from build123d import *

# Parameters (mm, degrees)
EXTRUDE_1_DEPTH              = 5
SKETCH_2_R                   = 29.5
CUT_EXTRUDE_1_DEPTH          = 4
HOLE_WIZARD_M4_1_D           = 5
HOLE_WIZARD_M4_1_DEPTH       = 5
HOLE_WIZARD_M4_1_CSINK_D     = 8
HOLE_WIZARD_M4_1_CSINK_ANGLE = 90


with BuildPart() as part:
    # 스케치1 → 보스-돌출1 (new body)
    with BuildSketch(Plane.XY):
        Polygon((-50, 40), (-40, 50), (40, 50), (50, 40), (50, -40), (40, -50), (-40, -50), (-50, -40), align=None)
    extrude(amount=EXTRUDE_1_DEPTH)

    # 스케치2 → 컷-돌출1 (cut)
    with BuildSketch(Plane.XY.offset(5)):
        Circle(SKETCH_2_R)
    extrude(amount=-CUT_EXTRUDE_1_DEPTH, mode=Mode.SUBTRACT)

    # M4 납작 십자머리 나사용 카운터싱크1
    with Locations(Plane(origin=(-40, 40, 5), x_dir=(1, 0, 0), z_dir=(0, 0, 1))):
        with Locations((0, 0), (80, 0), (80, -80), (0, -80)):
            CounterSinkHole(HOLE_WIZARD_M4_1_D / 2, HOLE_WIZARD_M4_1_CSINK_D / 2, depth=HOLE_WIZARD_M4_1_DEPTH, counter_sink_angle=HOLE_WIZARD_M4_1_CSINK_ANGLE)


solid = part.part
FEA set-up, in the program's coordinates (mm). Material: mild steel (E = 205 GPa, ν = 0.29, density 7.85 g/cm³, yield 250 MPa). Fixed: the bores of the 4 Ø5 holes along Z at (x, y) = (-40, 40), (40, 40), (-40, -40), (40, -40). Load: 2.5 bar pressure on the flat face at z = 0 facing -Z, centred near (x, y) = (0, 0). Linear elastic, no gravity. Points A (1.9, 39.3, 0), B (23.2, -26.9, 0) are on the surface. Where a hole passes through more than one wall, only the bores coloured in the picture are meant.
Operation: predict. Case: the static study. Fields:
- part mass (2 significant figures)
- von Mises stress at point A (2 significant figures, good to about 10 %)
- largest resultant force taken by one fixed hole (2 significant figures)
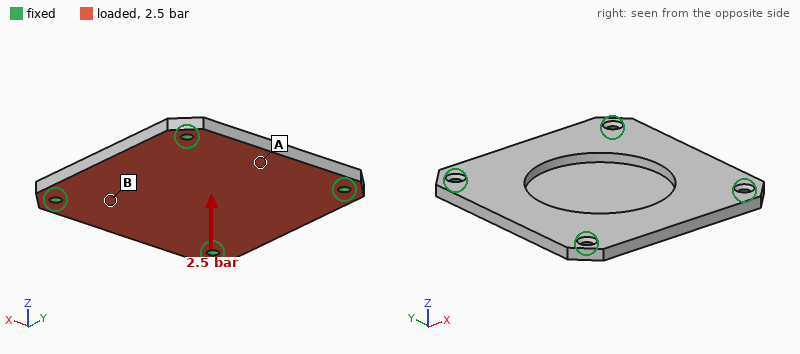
300 g
25 MPa
640 N
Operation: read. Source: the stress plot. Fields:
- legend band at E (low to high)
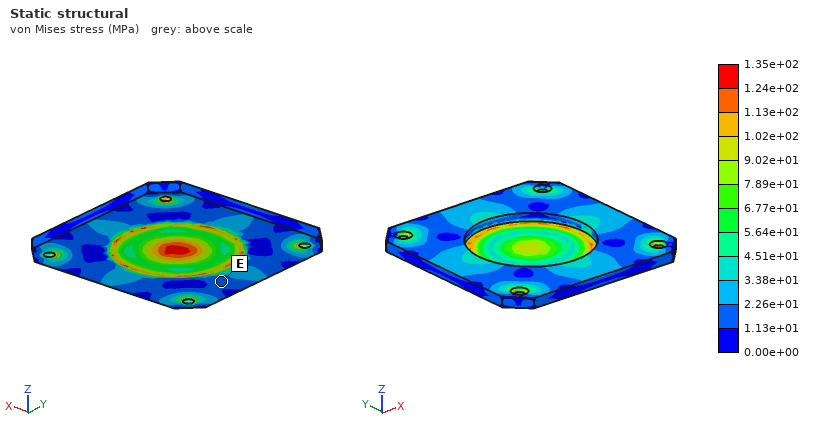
1.13e+01 to 2.26e+01 MPa
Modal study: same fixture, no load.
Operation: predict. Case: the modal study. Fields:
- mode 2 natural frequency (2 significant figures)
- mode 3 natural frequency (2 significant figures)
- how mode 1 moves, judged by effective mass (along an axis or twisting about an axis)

3800 Hz
3900 Hz
along Z
